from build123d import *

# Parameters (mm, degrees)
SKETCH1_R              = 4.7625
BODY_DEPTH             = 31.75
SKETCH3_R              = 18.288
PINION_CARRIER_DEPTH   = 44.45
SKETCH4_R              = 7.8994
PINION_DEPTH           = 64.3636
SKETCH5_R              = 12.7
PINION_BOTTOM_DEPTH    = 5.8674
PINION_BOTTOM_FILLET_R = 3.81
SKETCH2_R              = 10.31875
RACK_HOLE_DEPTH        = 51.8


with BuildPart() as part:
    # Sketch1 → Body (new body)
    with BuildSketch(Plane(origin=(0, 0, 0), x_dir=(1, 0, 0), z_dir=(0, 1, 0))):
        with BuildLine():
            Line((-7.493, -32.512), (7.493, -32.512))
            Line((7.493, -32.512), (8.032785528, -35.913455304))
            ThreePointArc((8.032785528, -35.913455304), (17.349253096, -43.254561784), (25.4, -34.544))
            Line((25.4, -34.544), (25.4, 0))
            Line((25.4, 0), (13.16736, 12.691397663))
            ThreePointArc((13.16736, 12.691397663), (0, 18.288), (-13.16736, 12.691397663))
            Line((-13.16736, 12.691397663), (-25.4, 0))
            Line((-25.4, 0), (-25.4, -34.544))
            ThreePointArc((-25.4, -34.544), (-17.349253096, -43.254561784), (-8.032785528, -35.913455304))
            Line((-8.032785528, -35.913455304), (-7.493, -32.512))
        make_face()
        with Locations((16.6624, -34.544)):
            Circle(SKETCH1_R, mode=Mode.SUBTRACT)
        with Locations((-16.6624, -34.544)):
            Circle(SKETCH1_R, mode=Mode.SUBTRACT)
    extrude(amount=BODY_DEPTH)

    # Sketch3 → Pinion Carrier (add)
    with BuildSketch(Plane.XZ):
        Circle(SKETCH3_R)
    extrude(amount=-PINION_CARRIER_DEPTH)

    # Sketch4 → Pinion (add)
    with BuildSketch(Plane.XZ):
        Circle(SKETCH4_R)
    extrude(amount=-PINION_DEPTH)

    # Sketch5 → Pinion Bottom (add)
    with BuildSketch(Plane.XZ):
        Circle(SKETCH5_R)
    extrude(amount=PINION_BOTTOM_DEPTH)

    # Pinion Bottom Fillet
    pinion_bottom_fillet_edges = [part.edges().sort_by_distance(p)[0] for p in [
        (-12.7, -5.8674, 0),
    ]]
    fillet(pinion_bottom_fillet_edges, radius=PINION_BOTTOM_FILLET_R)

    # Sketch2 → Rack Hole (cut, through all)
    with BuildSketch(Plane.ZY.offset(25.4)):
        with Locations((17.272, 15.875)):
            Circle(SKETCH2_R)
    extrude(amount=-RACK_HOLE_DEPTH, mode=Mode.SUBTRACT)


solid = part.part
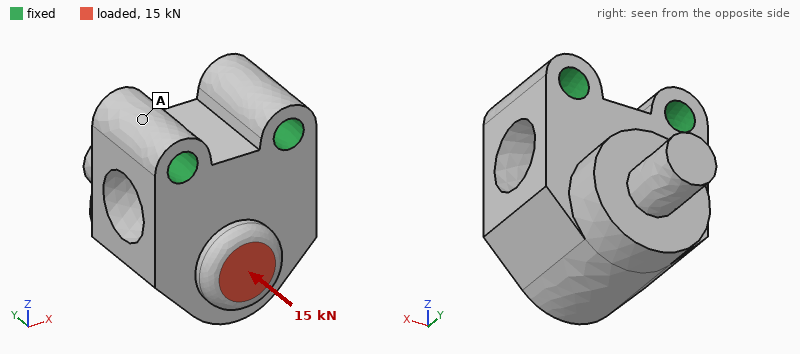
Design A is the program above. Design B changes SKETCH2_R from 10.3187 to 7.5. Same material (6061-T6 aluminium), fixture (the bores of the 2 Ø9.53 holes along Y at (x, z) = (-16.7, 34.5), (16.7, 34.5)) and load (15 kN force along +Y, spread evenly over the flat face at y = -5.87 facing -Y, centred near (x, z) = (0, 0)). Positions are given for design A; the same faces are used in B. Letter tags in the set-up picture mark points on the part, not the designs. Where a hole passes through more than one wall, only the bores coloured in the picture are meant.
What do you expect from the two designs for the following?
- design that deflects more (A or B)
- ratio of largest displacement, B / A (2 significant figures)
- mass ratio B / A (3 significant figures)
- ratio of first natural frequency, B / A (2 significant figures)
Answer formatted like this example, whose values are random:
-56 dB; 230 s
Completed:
A; 0.66; 1.10; 1.2
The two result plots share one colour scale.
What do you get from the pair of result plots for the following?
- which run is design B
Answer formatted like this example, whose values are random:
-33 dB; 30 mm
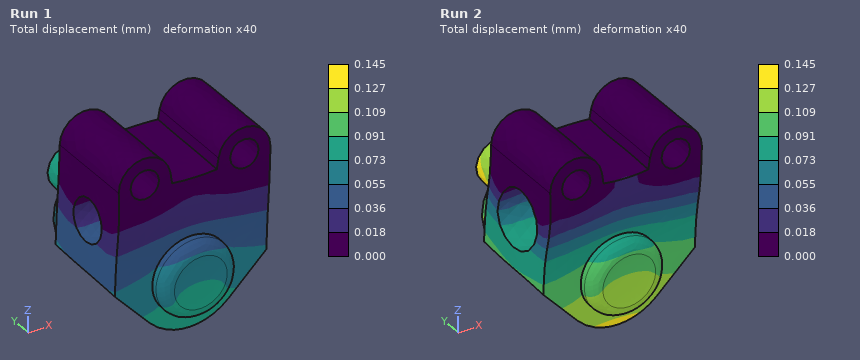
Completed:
Run 1
